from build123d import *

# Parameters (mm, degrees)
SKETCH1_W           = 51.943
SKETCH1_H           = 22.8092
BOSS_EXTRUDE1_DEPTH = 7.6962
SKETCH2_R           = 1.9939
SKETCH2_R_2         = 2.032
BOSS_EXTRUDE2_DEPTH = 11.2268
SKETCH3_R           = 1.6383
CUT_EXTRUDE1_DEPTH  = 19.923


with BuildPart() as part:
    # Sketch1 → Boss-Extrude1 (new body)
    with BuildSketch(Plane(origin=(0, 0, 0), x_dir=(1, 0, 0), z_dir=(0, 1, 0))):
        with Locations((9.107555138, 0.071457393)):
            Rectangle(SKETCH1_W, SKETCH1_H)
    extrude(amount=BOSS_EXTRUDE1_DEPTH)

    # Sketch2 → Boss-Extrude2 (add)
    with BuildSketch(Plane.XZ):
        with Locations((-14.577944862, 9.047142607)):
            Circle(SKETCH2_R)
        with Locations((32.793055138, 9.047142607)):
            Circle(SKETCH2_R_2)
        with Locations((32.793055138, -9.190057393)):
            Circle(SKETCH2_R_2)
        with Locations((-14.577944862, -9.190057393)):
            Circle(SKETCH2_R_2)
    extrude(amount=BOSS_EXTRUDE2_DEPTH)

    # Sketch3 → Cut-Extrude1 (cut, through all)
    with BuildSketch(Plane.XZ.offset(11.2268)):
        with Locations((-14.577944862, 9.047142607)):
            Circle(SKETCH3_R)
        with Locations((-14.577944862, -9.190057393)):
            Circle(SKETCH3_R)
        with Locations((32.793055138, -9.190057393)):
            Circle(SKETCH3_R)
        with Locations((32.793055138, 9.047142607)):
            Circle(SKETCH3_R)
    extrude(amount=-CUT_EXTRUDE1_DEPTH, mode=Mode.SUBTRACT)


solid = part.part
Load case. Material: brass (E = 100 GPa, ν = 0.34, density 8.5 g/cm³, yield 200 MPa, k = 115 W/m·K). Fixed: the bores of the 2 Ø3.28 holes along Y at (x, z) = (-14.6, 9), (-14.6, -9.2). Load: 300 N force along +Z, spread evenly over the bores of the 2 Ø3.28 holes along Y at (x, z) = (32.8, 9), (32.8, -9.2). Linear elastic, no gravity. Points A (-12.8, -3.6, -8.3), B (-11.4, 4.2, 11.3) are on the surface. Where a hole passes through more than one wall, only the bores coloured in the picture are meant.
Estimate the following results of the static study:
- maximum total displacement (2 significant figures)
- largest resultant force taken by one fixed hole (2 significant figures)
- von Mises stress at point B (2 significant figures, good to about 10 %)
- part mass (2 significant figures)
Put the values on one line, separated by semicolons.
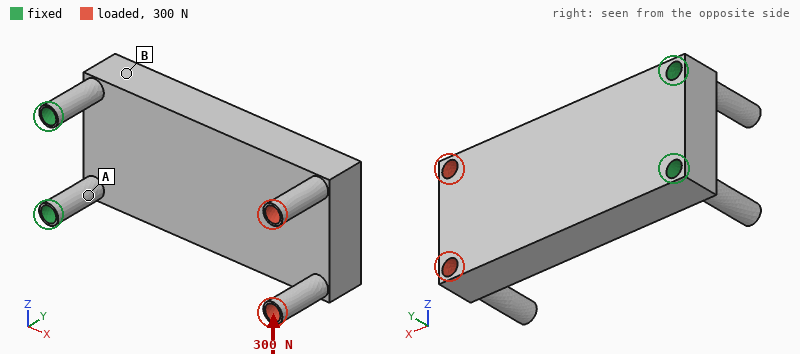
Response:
65 µm; 780 N; 19 MPa; 77 g
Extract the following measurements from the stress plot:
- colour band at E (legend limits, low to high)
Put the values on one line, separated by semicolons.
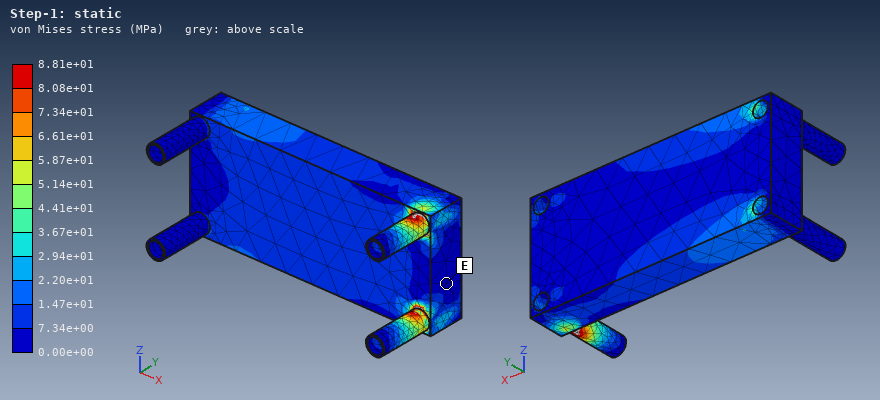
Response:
0.00e+00 to 7.34e+00 MPa
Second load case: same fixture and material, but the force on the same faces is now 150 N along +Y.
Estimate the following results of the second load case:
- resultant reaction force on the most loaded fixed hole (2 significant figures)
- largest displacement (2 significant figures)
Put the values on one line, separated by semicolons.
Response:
75 N; 80 µm
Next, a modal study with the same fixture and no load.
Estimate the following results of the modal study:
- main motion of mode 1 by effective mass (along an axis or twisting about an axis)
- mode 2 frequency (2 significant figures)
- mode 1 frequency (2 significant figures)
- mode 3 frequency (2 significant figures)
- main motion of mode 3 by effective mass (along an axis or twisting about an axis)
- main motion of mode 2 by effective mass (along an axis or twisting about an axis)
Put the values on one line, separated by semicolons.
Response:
along Y; 4600 Hz; 1600 Hz; 6400 Hz; twisting about X; along Z
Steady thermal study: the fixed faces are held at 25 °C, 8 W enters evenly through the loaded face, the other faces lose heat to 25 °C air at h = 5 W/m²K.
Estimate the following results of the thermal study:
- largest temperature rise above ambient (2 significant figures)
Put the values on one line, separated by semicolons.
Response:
48 K
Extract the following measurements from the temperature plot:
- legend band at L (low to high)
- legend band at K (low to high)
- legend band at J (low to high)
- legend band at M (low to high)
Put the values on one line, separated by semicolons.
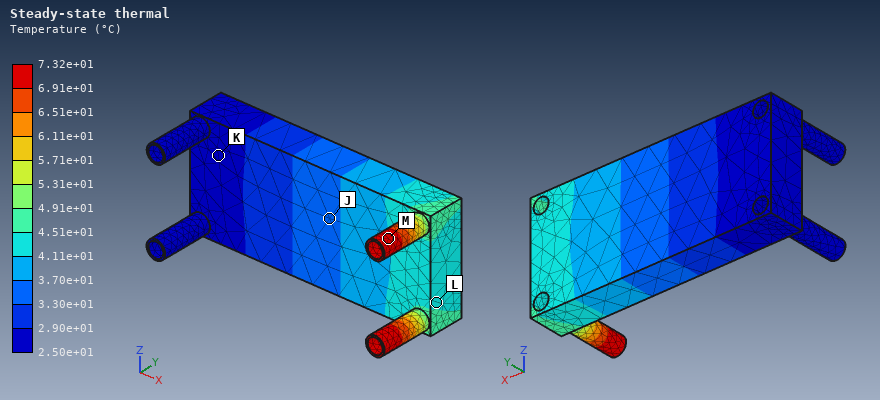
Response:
4.11e+01 to 4.51e+01 °C; 2.50e+01 to 2.90e+01 °C; 3.30e+01 to 3.70e+01 °C; 6.91e+01 to 7.32e+01 °C
